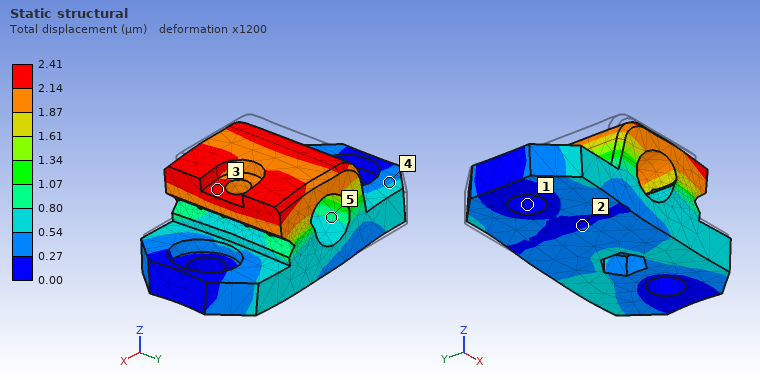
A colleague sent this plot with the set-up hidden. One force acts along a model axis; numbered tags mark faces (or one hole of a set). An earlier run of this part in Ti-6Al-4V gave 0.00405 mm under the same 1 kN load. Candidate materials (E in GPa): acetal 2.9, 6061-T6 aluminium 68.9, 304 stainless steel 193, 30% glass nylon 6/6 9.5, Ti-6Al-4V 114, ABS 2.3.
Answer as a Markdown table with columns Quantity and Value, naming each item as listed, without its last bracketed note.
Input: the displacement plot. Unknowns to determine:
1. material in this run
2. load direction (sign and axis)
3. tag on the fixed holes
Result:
| Quantity | Value |
|---|---|
| material in this run | 304 stainless steel |
| load direction | +X |
| tag on the fixed holes | 1 |
